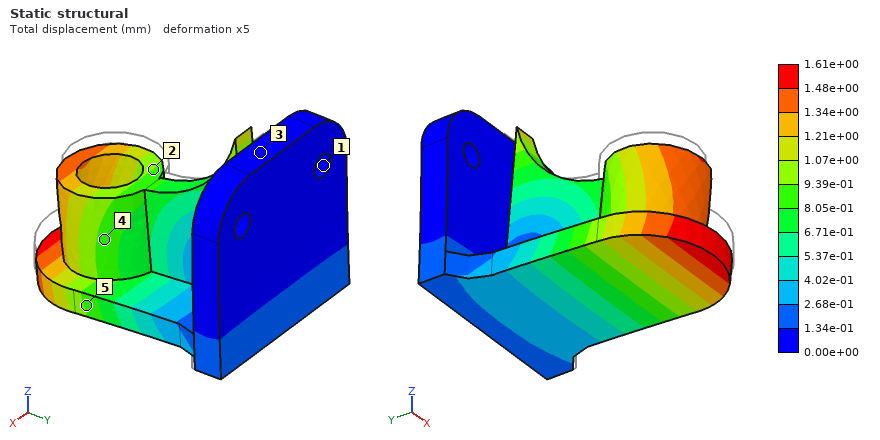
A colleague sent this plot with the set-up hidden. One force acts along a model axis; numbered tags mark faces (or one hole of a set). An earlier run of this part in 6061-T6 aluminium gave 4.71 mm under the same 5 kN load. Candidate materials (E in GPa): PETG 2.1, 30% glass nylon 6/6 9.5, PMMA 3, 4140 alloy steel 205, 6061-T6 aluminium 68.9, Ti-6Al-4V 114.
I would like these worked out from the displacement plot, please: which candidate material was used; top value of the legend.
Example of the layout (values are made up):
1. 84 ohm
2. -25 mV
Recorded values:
1. 4140 alloy steel
2. 1.61e+00 mm
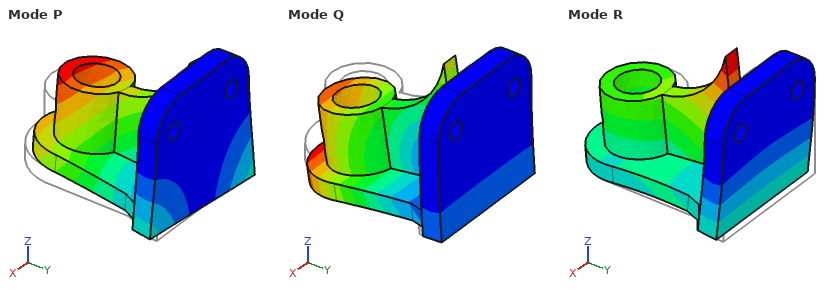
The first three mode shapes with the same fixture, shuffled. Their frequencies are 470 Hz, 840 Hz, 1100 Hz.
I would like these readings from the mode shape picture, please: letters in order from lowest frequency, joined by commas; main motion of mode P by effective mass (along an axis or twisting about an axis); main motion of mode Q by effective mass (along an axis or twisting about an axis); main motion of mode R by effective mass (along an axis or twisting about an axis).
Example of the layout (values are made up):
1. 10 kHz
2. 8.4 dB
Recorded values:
1. Q, P, R
2. along X
3. along Z
4. along Y
